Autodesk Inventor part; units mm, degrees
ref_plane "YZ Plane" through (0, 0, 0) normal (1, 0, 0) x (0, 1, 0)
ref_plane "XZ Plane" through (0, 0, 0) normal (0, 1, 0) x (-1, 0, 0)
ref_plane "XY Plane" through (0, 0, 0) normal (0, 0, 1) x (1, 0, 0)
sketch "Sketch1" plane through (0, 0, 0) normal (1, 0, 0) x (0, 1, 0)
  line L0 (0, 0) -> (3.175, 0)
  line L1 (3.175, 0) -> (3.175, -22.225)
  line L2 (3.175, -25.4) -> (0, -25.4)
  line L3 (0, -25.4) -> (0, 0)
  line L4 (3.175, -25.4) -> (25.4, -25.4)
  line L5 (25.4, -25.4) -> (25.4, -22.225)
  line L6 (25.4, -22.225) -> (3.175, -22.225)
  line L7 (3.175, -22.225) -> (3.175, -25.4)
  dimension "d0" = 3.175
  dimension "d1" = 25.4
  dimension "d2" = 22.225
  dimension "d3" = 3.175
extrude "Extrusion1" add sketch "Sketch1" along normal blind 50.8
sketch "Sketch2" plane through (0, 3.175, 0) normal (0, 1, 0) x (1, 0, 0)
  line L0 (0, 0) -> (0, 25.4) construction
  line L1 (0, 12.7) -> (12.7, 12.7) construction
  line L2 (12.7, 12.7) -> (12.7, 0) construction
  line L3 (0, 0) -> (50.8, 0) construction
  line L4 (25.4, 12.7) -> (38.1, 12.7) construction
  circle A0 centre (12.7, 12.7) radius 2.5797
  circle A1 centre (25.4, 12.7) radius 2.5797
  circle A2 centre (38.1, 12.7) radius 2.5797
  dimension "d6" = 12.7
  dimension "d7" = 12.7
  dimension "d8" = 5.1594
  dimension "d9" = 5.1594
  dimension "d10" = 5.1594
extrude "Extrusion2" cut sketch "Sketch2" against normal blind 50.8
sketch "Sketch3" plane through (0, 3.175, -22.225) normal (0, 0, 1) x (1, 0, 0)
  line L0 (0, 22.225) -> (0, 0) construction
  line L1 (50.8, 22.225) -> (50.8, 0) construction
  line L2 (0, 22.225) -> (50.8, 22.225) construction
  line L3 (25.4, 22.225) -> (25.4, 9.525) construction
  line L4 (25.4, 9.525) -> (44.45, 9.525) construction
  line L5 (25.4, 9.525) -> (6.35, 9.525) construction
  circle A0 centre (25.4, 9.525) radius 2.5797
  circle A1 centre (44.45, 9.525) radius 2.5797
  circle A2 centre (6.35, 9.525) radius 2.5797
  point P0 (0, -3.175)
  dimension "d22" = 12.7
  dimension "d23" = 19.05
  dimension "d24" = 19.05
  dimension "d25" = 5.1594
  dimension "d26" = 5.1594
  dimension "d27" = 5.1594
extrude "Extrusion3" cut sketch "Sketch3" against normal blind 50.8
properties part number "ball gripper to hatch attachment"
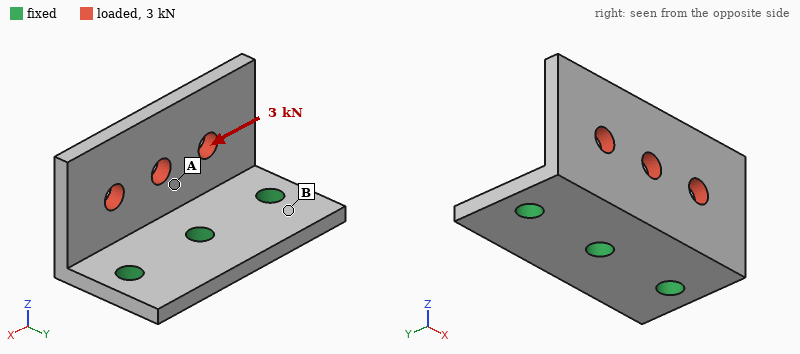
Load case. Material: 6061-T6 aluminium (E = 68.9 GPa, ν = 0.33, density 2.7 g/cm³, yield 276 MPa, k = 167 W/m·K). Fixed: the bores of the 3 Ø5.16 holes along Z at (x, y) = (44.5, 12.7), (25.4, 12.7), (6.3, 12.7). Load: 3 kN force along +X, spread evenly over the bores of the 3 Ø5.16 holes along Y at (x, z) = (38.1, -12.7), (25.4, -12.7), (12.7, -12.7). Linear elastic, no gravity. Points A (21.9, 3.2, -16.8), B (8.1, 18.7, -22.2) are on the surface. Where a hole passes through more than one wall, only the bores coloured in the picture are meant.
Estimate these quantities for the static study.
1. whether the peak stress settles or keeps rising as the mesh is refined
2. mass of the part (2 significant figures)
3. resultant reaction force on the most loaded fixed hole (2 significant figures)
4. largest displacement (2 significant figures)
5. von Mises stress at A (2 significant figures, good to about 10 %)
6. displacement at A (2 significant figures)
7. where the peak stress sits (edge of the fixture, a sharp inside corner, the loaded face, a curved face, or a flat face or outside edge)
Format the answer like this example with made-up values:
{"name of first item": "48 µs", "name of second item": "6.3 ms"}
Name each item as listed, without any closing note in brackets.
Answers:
{"whether the peak stress settles or keeps rising as the mesh is refined": "keeps rising", "mass of the part": "20 g", "resultant reaction force on the most loaded fixed hole": "1.4 kN", "largest displacement": "0.17 mm", "von Mises stress at A": "69 MPa", "displacement at A": "0.039 mm", "where the peak stress sits": "edge of the fixture"}
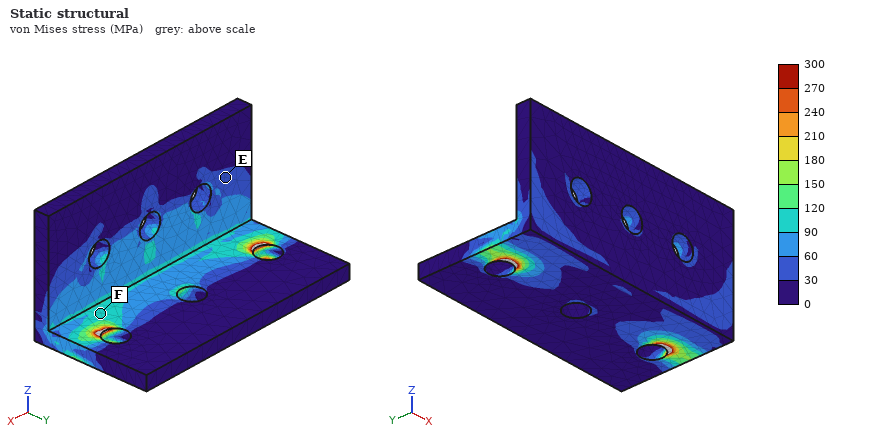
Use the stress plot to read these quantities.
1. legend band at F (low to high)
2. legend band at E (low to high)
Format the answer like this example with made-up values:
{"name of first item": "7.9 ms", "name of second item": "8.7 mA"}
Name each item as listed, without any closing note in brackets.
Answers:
{"legend band at F": "90 to 120 MPa", "legend band at E": "30 to 60 MPa"}
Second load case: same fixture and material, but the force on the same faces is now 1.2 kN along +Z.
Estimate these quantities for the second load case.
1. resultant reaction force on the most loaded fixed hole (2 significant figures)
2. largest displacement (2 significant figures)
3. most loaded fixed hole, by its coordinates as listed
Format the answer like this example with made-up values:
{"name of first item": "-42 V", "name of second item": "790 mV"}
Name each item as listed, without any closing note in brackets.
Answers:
{"resultant reaction force on the most loaded fixed hole": "450 N", "largest displacement": "0.16 mm", "most loaded fixed hole, by its coordinates as listed": "(25.4, 12.7)"}
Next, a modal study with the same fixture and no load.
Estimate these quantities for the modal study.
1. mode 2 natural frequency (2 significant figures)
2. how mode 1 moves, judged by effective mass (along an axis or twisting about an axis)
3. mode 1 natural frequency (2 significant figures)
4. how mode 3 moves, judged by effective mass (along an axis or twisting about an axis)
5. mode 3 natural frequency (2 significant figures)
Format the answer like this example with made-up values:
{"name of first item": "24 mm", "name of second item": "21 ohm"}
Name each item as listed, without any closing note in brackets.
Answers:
{"mode 2 natural frequency": "4900 Hz", "how mode 1 moves, judged by effective mass": "along Y", "mode 1 natural frequency": "2900 Hz", "how mode 3 moves, judged by effective mass": "along X", "mode 3 natural frequency": "9100 Hz"}
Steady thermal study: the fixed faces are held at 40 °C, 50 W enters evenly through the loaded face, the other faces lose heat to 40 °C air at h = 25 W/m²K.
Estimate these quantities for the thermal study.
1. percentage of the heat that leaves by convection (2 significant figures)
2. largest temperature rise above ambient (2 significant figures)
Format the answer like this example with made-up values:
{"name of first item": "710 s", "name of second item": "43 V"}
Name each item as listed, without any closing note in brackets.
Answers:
{"percentage of the heat that leaves by convection": "4.9 %", "largest temperature rise above ambient": "45 K"}
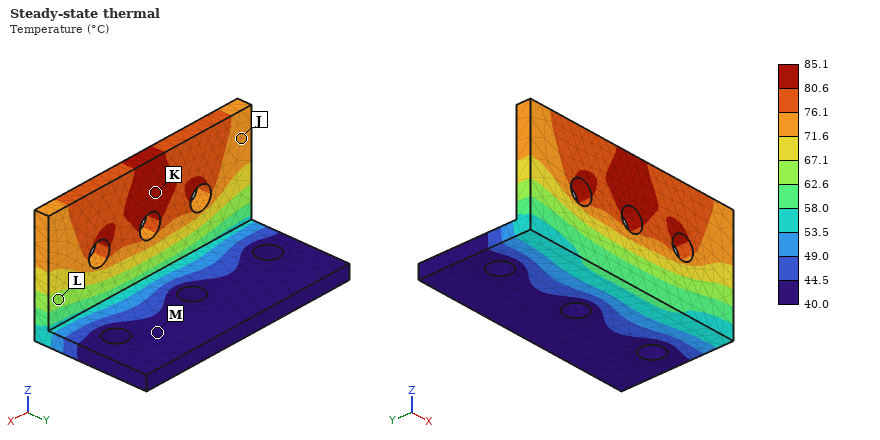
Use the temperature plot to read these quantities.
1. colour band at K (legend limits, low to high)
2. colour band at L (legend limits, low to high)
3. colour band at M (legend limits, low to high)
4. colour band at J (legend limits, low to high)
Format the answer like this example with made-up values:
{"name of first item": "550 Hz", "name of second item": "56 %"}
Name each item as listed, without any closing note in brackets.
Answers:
{"colour band at K": "80.6 to 85.1 °C", "colour band at L": "62.6 to 67.1 °C", "colour band at M": "40.0 to 44.5 °C", "colour band at J": "71.6 to 76.1 °C"}
